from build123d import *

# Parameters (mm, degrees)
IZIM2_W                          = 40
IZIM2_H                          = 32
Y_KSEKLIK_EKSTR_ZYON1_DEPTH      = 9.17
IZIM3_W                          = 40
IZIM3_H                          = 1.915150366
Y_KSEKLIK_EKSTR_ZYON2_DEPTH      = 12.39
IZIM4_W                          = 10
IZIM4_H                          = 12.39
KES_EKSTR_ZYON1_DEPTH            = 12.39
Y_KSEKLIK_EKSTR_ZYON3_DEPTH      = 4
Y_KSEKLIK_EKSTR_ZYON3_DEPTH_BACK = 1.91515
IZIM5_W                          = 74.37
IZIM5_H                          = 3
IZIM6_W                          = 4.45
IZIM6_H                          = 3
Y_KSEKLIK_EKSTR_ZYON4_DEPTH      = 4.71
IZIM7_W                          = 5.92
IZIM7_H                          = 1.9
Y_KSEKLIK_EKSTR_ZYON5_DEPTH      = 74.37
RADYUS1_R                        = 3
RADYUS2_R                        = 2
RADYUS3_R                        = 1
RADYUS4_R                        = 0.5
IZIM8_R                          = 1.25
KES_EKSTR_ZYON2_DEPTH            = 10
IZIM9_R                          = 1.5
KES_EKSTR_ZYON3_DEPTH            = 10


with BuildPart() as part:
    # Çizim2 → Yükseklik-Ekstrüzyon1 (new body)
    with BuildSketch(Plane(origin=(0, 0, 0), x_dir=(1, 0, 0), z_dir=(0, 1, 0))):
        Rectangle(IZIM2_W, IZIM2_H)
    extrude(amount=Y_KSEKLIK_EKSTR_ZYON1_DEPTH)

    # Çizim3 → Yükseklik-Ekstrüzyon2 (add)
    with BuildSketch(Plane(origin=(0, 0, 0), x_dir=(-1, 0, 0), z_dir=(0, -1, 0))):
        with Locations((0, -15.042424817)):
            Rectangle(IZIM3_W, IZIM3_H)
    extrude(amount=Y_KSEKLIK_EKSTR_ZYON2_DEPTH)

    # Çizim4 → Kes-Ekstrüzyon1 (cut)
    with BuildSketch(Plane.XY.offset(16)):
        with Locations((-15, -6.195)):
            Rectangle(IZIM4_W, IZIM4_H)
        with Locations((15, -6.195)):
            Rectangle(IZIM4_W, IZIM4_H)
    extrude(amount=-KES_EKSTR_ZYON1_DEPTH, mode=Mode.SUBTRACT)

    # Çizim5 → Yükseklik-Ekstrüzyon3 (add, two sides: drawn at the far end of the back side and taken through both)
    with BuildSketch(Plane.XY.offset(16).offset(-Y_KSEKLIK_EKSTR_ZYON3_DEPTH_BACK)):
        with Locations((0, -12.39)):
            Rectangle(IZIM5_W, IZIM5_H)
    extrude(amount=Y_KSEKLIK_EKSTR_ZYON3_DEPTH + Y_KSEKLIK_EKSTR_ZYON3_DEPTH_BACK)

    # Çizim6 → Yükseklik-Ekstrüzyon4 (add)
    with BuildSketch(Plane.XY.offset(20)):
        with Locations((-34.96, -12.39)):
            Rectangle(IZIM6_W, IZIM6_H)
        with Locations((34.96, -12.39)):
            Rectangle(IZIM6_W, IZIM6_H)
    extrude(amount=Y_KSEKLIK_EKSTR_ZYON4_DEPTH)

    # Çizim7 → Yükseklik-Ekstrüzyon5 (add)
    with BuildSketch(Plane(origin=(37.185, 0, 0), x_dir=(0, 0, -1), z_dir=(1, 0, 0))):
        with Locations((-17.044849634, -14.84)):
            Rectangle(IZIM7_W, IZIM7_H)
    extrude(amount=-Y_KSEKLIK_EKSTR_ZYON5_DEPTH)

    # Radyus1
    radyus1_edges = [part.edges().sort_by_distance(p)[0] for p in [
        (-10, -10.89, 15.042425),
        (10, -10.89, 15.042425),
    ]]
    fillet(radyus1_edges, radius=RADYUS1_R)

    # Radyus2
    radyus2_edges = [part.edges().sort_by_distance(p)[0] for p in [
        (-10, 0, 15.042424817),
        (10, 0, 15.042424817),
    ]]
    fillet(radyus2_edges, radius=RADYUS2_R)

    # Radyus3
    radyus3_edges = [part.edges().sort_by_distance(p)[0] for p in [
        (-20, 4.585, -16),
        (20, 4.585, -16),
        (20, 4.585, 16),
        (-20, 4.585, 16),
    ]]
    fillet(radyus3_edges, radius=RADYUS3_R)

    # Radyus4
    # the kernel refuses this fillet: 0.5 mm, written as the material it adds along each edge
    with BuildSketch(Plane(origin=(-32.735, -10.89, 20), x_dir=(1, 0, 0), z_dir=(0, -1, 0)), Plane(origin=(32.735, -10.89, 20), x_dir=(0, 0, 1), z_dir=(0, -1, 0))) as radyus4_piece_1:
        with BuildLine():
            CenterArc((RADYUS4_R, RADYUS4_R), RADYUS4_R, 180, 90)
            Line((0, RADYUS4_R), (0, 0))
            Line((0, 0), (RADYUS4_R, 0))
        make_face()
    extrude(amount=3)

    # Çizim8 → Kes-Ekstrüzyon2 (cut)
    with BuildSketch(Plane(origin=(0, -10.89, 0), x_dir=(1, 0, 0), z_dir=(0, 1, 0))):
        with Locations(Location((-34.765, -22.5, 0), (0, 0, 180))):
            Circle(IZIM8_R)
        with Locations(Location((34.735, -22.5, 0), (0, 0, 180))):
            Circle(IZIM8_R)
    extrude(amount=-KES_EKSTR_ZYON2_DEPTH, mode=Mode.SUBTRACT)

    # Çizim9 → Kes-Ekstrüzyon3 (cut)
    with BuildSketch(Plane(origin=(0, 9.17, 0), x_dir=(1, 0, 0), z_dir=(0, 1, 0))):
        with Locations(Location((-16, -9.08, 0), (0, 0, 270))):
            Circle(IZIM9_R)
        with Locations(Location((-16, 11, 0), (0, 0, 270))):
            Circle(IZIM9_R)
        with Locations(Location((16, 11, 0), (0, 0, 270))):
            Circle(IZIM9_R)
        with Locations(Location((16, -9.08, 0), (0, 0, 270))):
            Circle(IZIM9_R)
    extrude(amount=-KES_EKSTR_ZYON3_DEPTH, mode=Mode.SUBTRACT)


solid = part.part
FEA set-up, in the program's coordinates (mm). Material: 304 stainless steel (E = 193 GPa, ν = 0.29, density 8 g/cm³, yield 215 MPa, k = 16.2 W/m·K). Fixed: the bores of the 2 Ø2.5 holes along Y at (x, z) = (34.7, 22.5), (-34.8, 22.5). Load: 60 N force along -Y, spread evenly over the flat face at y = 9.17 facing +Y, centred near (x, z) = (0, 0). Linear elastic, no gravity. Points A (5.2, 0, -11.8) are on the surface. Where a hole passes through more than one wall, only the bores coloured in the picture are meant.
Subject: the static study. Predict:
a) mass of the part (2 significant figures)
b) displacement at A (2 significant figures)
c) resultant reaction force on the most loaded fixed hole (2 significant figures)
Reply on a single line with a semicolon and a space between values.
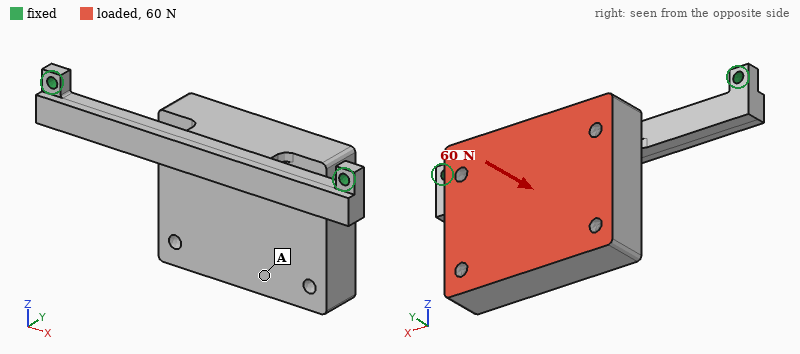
110 g; 0.21 mm; 34 N
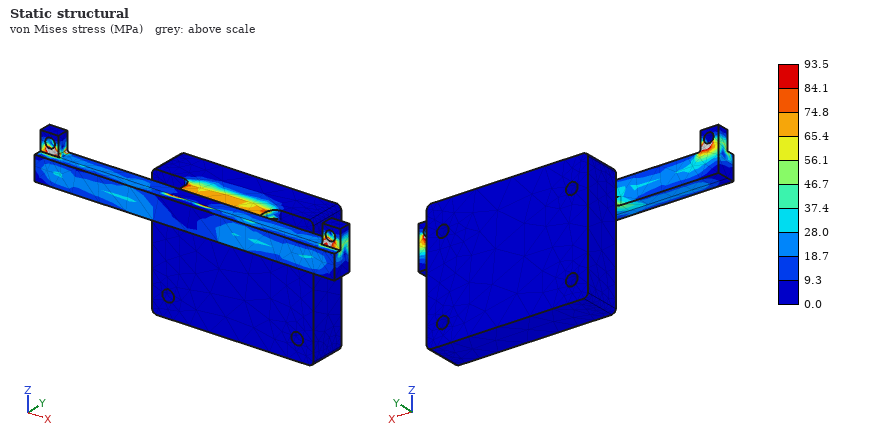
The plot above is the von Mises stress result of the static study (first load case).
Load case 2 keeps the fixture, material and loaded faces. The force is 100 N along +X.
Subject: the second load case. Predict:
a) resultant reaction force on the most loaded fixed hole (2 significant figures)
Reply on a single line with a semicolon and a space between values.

70 N
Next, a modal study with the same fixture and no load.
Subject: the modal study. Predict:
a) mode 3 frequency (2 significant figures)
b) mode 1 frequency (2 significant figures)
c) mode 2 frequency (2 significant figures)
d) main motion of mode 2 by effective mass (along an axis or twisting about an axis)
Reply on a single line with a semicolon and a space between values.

1100 Hz; 270 Hz; 620 Hz; along X
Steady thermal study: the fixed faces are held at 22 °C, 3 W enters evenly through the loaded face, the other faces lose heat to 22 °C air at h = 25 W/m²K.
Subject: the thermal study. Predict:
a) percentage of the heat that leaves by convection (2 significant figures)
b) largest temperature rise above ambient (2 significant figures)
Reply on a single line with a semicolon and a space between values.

90 %; 32 K
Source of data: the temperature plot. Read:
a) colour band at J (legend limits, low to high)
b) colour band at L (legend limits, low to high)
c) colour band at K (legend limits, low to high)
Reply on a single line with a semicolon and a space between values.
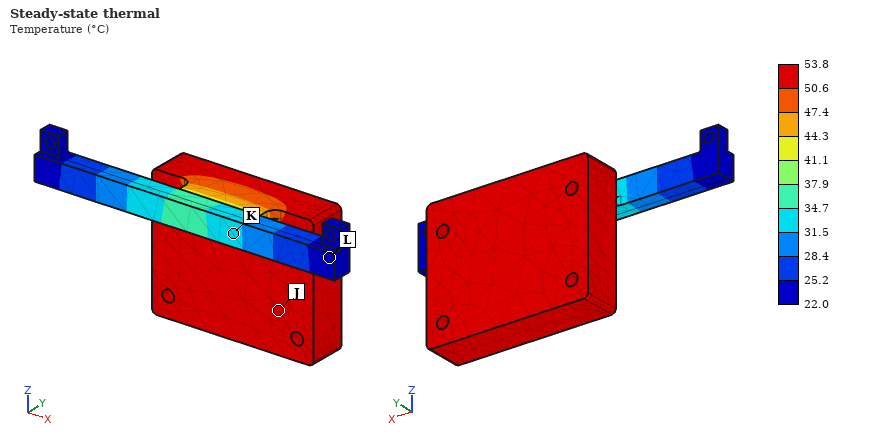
50.6 to 53.8 °C; 22.0 to 25.2 °C; 31.5 to 34.7 °C
